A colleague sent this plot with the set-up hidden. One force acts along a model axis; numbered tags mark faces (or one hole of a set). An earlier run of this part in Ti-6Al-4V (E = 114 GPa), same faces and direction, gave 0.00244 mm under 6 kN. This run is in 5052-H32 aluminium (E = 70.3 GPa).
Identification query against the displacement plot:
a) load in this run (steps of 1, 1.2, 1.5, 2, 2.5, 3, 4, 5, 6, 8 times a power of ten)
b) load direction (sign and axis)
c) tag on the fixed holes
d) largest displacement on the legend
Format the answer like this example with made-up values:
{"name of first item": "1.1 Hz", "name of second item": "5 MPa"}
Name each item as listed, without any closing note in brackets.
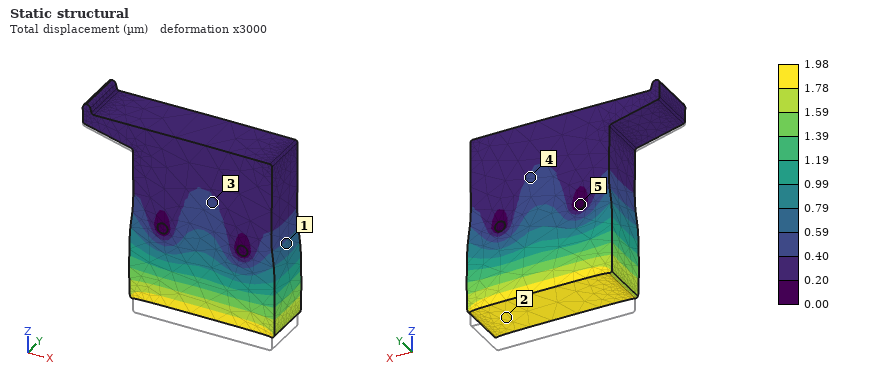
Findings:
{"load in this run": "3 kN", "load direction": "+Z", "tag on the fixed holes": "5", "largest displacement on the legend": "1.98 µm"}
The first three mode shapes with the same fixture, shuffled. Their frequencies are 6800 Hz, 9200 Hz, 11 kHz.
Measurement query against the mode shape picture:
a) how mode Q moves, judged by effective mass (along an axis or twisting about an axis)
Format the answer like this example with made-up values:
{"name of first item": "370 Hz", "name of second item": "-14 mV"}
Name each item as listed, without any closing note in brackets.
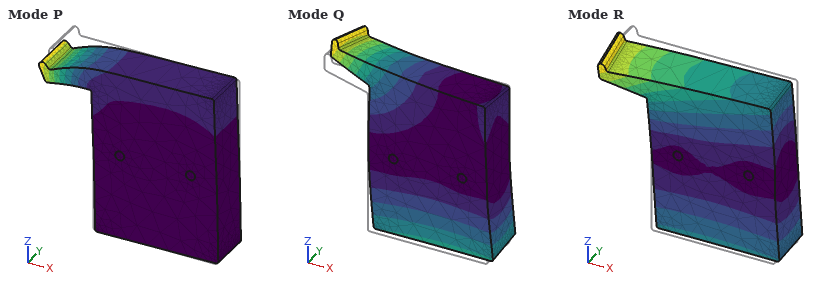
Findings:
{"how mode Q moves, judged by effective mass": "along Y"}
